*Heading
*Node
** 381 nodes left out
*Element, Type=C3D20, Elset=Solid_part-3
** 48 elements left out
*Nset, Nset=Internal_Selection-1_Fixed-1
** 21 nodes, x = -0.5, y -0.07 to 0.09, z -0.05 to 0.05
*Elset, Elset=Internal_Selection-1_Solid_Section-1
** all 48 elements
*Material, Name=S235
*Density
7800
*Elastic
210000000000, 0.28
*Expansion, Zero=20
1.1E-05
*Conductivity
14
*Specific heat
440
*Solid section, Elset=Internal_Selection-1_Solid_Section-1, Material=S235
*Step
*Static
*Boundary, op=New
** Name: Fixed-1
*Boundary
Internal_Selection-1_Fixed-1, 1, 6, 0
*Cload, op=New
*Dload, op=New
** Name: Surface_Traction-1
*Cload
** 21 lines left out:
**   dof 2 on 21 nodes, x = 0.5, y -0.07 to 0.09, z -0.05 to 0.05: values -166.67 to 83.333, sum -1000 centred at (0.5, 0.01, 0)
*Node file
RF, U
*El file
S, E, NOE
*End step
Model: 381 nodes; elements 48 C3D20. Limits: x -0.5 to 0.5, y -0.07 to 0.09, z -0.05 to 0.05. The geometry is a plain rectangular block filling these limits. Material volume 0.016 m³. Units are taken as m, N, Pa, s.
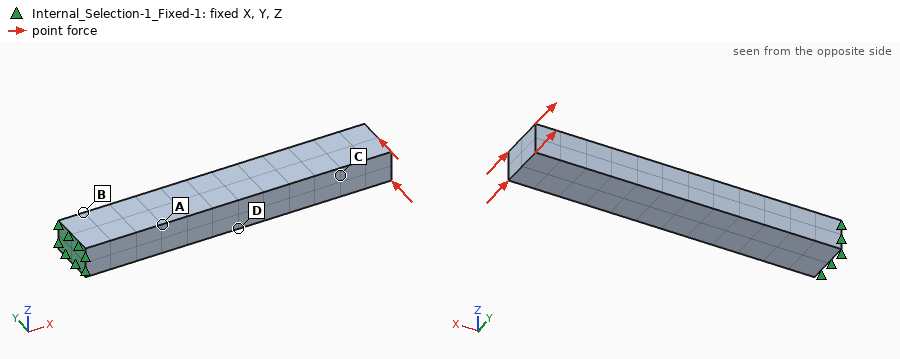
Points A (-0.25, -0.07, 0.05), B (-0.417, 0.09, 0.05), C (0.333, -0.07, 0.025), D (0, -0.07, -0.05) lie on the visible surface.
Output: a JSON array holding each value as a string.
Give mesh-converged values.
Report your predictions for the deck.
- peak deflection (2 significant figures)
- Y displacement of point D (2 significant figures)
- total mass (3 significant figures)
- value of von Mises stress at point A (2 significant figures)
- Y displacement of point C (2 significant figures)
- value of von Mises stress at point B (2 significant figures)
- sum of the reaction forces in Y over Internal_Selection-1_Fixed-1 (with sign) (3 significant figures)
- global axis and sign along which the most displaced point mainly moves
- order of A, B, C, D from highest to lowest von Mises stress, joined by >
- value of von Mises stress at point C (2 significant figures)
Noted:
["4.7e-05 m", "-1.5e-05 m", "125 kg", "1.8e+06 Pa", "-3.5e-05 m", "2.1e+06 Pa", "1000 N", "-Y", "B > A > D > C", "3.9e+05 Pa"]
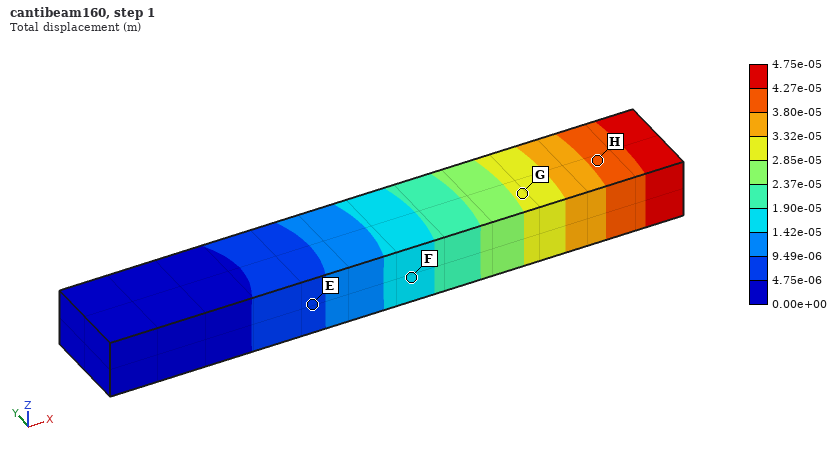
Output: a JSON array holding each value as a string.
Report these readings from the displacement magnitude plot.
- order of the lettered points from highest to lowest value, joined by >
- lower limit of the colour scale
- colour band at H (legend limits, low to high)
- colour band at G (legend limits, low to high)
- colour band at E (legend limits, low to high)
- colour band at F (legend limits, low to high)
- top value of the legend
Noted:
["H > G > F > E", "0.00e+00 m", "3.80e-05 to 4.27e-05 m", "2.85e-05 to 3.32e-05 m", "4.75e-06 to 9.49e-06 m", "1.42e-05 to 1.90e-05 m", "4.75e-05 m"]
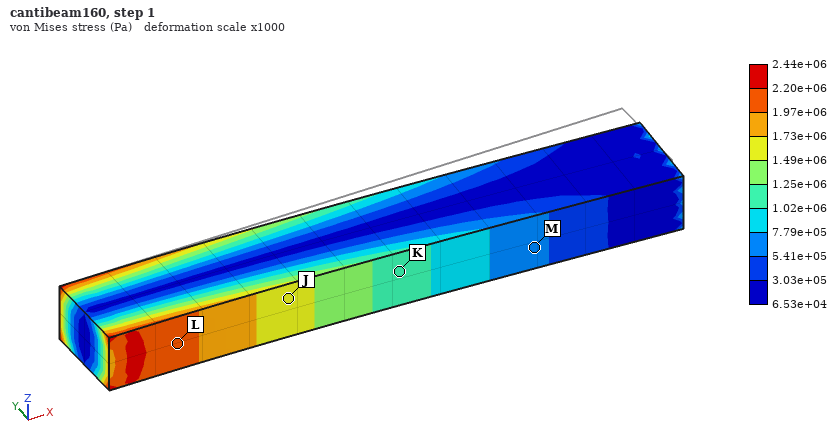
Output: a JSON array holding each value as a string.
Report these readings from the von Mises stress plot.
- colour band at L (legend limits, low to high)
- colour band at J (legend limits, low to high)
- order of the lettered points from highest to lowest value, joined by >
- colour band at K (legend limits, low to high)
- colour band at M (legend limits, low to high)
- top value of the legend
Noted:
["1.97e+06 to 2.20e+06 Pa", "1.49e+06 to 1.73e+06 Pa", "L > J > K > M", "1.02e+06 to 1.25e+06 Pa", "5.41e+05 to 7.79e+05 Pa", "2.44e+06 Pa"]
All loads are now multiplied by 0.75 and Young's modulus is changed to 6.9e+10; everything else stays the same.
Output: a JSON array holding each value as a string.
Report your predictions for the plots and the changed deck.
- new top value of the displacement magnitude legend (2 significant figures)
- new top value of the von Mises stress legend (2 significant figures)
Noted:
["1.1e-04 m", "1.8e+06 Pa"]
